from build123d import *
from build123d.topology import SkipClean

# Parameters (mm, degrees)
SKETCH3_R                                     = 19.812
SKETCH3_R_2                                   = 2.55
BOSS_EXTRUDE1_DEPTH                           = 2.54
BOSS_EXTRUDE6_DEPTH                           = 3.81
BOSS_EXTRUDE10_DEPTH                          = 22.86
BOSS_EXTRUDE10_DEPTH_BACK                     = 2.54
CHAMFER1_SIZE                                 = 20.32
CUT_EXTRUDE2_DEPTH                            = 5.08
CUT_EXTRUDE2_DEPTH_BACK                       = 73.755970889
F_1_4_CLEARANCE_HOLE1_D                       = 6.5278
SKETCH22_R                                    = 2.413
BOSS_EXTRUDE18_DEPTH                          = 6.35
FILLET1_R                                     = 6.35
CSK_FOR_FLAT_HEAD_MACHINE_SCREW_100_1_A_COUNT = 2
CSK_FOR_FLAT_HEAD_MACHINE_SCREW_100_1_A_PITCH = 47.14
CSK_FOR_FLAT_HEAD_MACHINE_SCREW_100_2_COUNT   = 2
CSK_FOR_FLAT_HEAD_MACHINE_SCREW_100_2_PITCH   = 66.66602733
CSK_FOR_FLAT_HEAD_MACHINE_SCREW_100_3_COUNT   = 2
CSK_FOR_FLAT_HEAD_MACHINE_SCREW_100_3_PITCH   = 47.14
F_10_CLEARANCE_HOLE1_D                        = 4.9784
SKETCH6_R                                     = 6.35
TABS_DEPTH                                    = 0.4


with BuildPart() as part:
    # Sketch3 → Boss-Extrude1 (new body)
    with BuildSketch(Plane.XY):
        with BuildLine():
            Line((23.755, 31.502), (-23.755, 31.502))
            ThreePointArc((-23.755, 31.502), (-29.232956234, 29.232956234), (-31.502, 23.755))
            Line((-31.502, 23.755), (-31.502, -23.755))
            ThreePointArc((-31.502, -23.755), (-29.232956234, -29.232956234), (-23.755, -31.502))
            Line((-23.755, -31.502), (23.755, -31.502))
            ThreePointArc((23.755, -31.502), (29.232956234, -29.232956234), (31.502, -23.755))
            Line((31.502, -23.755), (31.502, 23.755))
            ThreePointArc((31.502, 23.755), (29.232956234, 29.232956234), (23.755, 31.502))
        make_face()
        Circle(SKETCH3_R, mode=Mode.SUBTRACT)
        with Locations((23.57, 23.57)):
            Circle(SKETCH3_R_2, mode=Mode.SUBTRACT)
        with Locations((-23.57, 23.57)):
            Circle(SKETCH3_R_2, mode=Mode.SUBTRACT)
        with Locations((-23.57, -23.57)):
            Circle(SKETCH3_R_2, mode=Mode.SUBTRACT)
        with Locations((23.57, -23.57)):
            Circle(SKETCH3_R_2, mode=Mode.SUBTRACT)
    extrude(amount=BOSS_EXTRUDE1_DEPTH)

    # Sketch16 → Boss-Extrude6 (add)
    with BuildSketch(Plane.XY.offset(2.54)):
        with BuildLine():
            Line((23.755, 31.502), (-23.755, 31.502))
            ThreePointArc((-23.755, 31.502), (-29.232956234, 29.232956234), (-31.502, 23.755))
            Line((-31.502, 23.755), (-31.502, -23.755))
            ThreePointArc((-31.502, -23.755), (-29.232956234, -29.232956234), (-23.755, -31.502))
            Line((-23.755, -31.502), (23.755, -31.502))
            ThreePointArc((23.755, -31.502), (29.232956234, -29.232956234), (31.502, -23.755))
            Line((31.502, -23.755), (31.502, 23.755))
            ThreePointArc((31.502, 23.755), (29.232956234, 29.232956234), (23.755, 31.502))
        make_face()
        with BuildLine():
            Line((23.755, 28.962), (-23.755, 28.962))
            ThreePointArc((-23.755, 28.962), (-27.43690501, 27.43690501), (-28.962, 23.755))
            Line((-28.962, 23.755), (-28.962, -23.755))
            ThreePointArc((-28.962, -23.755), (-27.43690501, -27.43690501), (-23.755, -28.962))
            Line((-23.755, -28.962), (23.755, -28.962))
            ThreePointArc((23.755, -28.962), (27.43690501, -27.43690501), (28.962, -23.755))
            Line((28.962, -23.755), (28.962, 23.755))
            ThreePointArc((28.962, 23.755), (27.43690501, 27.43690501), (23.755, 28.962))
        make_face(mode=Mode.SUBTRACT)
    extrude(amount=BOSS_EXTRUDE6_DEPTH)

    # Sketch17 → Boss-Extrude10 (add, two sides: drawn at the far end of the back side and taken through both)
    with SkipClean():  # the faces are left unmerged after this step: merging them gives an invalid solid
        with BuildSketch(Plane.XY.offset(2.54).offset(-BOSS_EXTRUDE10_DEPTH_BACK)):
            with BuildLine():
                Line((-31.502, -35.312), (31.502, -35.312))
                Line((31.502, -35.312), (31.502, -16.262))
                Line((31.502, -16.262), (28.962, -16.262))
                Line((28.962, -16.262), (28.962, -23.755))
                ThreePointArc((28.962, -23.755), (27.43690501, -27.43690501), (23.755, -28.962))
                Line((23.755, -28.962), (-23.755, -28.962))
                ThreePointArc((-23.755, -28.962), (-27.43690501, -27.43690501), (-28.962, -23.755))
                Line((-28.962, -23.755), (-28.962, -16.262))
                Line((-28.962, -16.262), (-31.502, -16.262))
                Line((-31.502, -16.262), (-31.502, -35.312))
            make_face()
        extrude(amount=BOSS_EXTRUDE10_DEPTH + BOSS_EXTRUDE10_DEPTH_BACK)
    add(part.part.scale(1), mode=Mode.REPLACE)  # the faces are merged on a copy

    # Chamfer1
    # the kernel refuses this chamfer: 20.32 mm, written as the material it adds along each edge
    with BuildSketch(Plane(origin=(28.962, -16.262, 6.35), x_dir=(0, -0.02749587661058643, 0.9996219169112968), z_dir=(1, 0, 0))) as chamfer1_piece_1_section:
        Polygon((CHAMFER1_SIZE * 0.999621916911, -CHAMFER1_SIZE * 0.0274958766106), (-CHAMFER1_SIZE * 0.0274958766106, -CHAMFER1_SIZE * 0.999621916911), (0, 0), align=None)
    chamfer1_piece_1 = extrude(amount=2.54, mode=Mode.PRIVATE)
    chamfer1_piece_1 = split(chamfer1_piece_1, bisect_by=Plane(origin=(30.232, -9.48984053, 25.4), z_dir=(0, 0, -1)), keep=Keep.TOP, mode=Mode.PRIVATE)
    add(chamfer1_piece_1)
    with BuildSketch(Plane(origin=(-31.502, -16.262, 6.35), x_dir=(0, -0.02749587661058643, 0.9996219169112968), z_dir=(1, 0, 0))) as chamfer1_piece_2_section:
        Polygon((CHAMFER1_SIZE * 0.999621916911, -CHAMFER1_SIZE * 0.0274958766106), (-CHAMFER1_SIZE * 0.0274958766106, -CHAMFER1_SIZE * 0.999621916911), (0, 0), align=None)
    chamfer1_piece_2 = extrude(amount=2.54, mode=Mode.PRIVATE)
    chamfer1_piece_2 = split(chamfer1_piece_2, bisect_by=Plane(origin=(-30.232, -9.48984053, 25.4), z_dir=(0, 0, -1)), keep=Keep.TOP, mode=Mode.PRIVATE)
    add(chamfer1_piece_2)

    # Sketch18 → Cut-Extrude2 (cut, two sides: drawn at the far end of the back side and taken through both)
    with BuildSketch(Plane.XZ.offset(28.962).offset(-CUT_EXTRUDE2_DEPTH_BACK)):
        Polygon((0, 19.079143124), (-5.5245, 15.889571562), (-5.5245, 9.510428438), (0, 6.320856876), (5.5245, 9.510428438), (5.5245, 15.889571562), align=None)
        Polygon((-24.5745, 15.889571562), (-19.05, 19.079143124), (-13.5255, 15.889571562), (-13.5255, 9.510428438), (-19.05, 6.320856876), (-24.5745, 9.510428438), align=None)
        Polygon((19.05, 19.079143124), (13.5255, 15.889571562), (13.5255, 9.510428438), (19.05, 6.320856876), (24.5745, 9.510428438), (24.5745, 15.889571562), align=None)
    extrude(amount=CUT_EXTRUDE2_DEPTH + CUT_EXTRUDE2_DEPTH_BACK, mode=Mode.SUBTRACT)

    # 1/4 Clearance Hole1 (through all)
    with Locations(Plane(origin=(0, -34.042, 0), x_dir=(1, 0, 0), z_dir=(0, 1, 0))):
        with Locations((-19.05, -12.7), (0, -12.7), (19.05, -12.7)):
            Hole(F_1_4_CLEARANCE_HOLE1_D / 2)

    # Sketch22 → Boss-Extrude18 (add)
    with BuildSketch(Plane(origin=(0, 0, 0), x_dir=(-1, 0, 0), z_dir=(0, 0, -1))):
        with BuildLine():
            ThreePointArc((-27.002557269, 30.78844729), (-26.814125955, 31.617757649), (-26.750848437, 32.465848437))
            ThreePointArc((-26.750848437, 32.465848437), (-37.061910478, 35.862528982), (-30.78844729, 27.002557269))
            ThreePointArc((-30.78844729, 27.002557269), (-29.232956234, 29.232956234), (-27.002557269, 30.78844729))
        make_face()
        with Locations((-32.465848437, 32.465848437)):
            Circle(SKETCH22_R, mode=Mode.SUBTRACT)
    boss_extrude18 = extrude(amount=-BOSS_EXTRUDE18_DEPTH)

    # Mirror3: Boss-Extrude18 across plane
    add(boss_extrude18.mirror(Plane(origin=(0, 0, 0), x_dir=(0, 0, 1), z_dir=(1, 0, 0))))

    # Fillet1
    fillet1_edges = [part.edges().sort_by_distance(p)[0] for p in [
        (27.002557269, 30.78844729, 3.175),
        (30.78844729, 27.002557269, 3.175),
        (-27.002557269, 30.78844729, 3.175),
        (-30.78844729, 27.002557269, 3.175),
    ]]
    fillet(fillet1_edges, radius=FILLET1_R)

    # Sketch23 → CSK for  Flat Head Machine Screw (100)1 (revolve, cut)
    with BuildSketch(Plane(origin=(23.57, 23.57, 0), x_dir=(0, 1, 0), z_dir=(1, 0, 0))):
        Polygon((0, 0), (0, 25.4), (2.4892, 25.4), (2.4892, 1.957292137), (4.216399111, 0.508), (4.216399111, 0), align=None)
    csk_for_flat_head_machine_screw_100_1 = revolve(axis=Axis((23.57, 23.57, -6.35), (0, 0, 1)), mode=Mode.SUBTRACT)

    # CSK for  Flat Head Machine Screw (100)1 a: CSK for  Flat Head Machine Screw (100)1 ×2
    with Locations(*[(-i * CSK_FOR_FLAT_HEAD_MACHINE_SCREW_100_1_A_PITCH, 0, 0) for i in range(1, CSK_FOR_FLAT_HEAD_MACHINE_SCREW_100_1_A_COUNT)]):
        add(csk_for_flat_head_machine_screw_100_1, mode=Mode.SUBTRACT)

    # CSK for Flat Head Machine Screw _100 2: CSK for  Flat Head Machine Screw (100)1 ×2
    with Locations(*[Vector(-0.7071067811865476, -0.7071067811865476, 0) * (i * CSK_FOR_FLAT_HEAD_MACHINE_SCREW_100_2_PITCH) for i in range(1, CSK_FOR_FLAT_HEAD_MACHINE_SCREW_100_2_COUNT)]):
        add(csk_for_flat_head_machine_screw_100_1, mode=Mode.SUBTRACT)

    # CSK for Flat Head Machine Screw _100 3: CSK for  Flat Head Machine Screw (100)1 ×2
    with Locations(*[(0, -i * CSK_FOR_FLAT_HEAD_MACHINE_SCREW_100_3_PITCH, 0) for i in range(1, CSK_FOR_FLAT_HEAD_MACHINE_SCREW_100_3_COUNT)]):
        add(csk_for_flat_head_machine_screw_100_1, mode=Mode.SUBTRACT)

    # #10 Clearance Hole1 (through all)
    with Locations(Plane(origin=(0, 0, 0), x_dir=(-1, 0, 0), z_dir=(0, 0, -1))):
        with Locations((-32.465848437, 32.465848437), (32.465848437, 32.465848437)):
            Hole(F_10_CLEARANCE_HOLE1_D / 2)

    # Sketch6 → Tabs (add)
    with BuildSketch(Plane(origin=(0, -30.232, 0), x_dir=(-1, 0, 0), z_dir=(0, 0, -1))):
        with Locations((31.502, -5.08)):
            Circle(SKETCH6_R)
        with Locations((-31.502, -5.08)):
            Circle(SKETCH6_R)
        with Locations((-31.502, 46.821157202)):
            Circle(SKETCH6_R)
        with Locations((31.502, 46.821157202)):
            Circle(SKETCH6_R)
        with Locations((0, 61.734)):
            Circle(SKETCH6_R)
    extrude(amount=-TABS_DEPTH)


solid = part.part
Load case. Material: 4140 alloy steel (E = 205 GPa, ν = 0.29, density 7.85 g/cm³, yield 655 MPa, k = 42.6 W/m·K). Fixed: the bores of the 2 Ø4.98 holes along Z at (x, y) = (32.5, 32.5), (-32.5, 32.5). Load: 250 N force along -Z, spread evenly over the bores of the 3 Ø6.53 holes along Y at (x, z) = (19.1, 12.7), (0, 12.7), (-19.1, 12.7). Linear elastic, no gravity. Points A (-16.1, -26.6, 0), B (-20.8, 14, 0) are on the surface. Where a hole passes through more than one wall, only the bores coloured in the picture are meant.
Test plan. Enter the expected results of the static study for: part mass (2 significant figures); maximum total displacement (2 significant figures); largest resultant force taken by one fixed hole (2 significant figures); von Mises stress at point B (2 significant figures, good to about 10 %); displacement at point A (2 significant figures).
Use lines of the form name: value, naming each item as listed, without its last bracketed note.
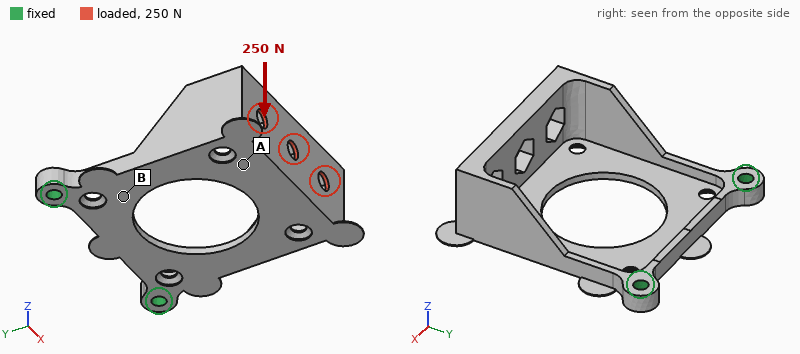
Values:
part mass: 160 g
maximum total displacement: 0.53 mm
largest resultant force taken by one fixed hole: 280 N
von Mises stress at point B: 84 MPa
displacement at point A: 0.39 mm
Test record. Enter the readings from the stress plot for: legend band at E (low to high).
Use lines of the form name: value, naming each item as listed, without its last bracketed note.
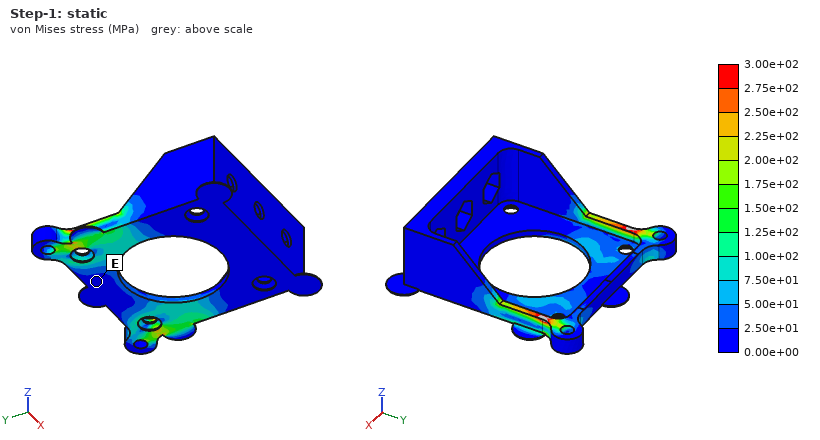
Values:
legend band at E: 0.00e+00 to 2.50e+01 MPa
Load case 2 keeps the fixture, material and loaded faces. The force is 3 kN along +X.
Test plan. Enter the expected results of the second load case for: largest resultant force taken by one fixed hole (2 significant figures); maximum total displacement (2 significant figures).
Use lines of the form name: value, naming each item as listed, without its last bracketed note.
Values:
largest resultant force taken by one fixed hole: 3.5 kN
maximum total displacement: 0.57 mm
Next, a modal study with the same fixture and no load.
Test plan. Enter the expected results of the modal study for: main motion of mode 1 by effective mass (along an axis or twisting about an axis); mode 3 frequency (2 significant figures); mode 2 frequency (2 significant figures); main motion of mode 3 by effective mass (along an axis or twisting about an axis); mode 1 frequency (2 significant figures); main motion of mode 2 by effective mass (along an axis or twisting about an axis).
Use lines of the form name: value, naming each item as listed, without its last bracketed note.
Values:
main motion of mode 1 by effective mass: along Z
mode 3 frequency: 3100 Hz
mode 2 frequency: 1100 Hz
main motion of mode 3 by effective mass: along X
mode 1 frequency: 390 Hz
main motion of mode 2 by effective mass: along X
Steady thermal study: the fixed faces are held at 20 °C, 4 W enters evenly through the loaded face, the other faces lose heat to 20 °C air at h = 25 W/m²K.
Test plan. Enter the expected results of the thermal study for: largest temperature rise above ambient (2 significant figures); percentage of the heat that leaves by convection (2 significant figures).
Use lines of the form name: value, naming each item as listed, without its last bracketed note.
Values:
largest temperature rise above ambient: 18 K
percentage of the heat that leaves by convection: 82 %
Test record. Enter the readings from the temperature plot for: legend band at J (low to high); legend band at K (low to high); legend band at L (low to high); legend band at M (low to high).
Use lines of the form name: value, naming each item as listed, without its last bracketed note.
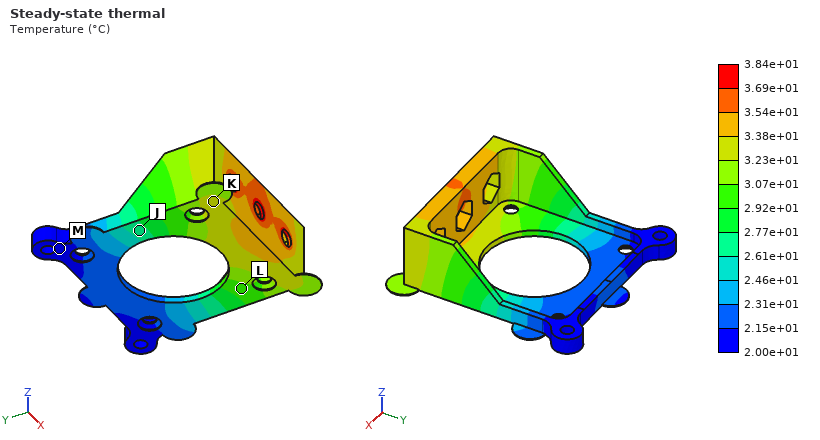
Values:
legend band at J: 2.61e+01 to 2.77e+01 °C
legend band at K: 3.23e+01 to 3.38e+01 °C
legend band at L: 2.92e+01 to 3.07e+01 °C
legend band at M: 2.00e+01 to 2.15e+01 °C
